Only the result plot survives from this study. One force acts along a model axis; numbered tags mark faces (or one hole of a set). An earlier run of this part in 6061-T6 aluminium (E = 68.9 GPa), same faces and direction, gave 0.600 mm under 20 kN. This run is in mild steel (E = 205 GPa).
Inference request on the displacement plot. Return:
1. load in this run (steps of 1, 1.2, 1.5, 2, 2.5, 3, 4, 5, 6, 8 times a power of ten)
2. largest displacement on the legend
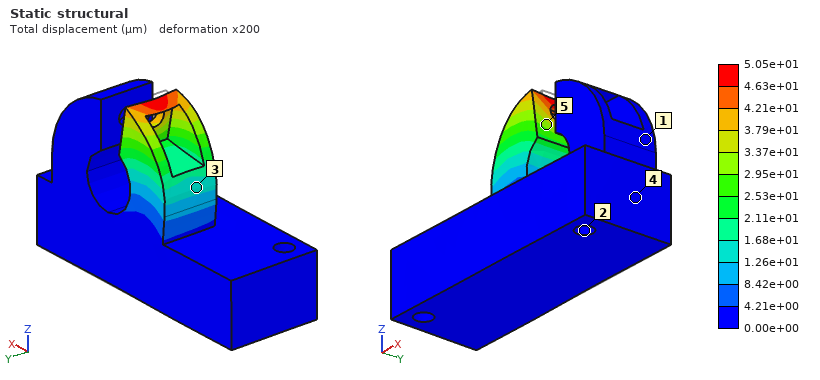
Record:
5 kN
5.05e+01 µm
